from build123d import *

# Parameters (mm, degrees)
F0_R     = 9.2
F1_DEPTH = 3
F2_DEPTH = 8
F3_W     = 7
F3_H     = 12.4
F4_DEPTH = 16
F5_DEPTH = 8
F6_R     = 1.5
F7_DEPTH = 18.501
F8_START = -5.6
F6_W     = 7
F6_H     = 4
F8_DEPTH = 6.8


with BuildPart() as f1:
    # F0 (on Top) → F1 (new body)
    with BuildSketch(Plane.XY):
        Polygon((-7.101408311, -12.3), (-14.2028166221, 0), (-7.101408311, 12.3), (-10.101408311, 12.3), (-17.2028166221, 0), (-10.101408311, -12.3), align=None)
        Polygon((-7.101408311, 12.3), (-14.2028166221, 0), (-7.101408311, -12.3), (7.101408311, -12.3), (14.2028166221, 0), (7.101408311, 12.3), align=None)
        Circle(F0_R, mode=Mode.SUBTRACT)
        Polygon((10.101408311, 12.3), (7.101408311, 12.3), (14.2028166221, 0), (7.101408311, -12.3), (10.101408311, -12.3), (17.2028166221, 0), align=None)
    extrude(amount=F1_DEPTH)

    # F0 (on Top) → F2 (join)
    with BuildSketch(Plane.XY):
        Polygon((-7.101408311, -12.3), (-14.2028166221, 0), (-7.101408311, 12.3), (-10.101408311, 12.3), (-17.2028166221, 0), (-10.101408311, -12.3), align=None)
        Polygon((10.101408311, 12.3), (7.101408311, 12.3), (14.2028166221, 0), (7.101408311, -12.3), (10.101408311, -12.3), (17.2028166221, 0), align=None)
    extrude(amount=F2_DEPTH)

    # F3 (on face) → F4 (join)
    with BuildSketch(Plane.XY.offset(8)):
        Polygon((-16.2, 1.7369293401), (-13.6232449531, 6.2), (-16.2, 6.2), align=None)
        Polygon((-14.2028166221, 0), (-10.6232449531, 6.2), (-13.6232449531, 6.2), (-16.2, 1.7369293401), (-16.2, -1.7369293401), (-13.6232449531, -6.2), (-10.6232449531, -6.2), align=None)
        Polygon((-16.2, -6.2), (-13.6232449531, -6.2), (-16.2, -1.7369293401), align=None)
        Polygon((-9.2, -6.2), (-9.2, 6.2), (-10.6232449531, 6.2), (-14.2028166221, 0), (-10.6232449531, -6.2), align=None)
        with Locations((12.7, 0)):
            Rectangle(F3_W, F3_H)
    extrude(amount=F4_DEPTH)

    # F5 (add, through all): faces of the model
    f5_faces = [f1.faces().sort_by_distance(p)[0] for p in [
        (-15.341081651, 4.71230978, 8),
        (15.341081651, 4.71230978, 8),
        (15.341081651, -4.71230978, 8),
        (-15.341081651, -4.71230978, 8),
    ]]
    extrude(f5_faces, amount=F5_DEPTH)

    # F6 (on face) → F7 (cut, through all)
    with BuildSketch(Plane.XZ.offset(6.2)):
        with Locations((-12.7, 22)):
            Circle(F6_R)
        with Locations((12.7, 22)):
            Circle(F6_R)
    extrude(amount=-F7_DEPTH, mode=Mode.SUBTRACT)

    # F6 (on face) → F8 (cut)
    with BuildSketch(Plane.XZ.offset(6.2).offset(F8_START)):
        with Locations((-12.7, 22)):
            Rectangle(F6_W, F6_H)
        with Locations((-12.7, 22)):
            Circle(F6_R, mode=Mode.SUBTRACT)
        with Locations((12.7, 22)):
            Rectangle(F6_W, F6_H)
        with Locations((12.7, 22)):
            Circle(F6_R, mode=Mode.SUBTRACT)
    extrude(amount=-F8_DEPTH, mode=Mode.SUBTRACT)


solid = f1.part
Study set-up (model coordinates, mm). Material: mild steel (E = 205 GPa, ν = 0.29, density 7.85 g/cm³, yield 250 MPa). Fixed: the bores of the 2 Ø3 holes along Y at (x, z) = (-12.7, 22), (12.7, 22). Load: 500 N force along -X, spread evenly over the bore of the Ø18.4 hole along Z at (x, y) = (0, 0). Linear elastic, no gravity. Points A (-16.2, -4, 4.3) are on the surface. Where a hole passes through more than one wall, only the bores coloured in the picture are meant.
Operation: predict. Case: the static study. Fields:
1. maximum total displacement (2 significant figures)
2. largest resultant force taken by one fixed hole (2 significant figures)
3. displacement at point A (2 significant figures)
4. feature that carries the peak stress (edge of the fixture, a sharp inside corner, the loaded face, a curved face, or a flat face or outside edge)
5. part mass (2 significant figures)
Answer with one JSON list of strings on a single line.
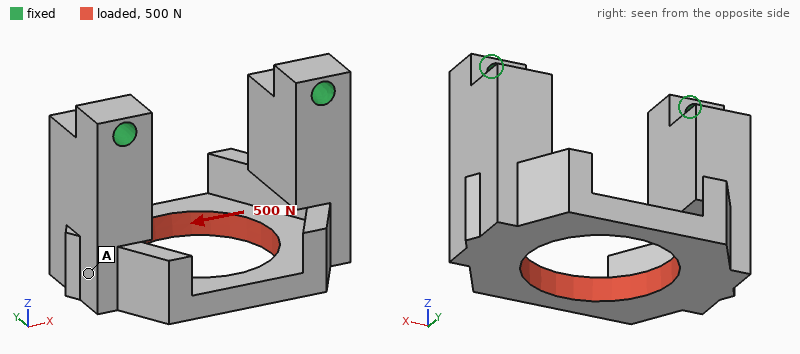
["17 µm", "270 N", "13 µm", "edge of the fixture", "35 g"]
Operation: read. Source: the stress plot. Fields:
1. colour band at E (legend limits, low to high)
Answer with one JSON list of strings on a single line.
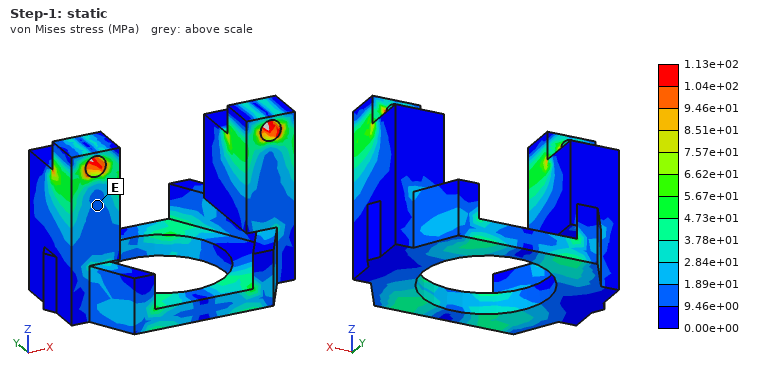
["9.46e+00 to 1.89e+01 MPa"]
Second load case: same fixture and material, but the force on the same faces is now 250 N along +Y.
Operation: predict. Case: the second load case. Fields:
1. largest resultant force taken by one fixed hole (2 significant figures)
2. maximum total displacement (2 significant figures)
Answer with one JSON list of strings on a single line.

["130 N", "14 µm"]
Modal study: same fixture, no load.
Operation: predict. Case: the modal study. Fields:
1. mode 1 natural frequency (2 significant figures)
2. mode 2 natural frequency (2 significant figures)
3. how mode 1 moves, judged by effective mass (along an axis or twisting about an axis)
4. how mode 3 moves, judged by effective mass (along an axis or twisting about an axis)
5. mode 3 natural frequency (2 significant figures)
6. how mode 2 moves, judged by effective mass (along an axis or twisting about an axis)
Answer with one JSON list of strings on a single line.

["5700 Hz", "6800 Hz", "along Y", "twisting about Z", "8600 Hz", "along X"]
